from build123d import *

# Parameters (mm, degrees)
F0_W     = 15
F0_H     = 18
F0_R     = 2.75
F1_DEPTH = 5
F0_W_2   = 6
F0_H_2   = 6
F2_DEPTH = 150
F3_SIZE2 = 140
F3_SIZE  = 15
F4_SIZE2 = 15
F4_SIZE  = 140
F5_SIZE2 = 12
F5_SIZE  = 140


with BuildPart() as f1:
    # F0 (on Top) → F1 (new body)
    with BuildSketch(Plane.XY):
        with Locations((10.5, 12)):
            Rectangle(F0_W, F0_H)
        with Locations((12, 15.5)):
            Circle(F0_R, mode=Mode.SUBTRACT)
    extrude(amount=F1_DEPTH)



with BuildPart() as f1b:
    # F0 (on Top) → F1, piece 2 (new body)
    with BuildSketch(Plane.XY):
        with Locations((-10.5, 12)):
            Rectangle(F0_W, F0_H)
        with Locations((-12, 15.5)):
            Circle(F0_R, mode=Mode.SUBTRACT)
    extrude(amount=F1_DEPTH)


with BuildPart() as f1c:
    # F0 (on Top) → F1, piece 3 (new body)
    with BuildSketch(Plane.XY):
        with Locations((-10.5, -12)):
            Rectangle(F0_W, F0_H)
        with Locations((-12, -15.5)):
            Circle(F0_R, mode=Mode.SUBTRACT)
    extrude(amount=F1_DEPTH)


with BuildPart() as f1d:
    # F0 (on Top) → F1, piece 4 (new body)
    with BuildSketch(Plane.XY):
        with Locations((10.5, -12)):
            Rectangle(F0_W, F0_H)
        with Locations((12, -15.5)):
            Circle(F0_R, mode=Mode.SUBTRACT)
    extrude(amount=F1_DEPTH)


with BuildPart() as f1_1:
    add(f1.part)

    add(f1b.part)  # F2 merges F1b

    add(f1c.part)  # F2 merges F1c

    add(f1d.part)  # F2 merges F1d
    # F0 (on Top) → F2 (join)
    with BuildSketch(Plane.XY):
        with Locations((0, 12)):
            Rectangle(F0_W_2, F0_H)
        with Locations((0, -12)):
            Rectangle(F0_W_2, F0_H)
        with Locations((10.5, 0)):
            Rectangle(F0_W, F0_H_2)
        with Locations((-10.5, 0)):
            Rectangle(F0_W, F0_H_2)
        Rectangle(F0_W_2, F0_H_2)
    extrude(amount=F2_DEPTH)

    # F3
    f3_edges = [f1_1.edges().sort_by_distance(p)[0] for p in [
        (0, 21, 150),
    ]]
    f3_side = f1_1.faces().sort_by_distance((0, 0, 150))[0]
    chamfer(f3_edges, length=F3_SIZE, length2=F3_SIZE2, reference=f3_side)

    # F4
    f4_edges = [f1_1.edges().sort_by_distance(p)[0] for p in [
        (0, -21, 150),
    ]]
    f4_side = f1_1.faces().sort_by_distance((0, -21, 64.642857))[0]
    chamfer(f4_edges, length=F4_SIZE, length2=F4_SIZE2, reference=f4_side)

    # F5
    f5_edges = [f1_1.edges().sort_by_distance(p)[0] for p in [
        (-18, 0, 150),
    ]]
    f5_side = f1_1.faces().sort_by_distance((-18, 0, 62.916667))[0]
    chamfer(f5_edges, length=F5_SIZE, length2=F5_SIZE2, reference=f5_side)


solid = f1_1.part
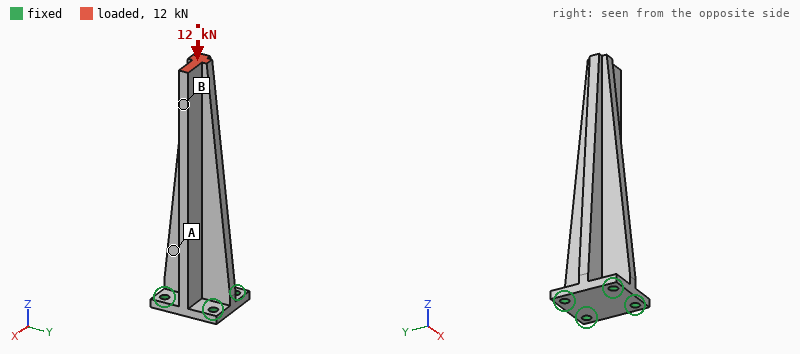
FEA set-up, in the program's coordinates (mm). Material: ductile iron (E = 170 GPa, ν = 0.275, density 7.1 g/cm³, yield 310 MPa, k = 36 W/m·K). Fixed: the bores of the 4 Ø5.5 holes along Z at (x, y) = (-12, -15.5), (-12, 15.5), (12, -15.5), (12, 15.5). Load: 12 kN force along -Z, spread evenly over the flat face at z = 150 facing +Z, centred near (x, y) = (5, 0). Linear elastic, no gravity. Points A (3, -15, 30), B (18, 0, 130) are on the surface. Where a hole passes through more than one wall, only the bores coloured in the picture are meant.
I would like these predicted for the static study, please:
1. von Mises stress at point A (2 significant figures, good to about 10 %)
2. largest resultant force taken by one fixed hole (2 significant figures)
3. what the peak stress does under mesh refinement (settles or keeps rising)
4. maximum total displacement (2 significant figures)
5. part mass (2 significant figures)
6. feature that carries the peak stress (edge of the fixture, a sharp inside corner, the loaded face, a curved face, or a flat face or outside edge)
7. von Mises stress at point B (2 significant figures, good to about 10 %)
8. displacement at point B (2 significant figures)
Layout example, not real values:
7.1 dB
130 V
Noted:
39 MPa
4.2 kN
keeps rising
0.27 mm
370 g
edge of the fixture
75 MPa
0.22 mm
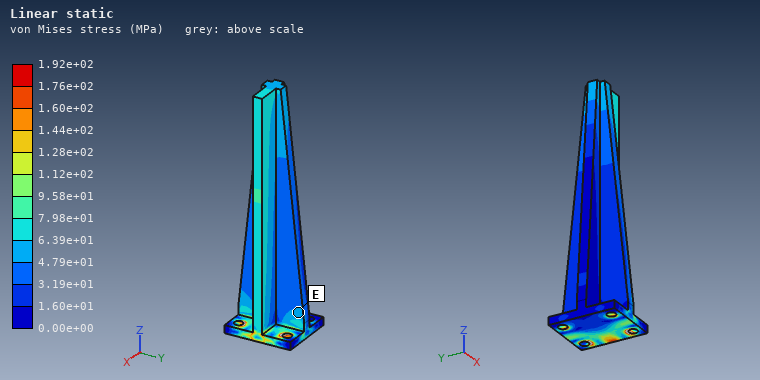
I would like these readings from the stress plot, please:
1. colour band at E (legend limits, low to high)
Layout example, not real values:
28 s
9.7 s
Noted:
4.79e+01 to 6.39e+01 MPa
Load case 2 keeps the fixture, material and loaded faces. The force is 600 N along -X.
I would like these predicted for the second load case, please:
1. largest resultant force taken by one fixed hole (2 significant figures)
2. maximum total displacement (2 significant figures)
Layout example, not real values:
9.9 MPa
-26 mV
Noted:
1.9 kN
0.36 mm
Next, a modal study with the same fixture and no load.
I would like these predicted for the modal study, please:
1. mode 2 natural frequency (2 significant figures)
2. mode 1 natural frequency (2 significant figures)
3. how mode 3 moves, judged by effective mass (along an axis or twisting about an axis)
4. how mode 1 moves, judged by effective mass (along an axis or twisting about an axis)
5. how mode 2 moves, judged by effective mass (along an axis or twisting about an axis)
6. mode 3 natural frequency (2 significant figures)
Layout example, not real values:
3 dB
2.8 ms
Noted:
1000 Hz
790 Hz
twisting about Z
along X
along Y
2800 Hz
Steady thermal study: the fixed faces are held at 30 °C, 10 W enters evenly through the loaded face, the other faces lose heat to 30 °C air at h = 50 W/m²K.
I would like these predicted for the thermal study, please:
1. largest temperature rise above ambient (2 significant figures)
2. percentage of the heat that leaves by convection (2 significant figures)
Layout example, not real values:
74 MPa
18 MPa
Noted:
56 K
93 %
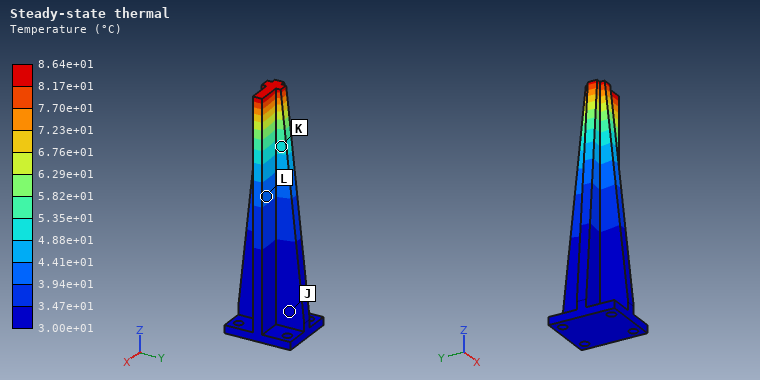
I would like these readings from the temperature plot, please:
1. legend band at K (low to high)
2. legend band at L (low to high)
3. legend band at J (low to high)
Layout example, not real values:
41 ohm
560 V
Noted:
4.88e+01 to 5.35e+01 °C
3.94e+01 to 4.41e+01 °C
3.00e+01 to 3.47e+01 °C
